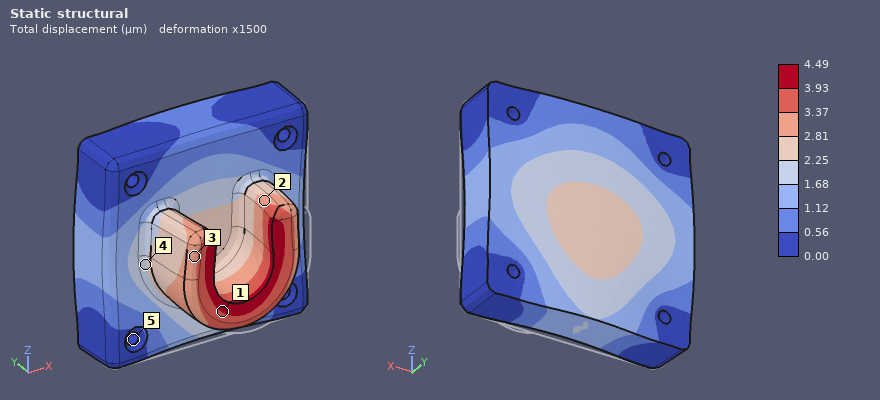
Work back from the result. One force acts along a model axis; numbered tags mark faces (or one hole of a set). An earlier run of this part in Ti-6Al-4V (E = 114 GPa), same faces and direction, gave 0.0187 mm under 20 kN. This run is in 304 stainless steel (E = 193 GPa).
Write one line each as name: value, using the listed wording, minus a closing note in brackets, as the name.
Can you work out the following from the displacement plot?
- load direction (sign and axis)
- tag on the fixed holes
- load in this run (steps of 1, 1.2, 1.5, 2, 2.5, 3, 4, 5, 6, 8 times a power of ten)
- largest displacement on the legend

load direction: +Y
tag on the fixed holes: 5
load in this run: 8 kN
largest displacement on the legend: 4.49 µm
